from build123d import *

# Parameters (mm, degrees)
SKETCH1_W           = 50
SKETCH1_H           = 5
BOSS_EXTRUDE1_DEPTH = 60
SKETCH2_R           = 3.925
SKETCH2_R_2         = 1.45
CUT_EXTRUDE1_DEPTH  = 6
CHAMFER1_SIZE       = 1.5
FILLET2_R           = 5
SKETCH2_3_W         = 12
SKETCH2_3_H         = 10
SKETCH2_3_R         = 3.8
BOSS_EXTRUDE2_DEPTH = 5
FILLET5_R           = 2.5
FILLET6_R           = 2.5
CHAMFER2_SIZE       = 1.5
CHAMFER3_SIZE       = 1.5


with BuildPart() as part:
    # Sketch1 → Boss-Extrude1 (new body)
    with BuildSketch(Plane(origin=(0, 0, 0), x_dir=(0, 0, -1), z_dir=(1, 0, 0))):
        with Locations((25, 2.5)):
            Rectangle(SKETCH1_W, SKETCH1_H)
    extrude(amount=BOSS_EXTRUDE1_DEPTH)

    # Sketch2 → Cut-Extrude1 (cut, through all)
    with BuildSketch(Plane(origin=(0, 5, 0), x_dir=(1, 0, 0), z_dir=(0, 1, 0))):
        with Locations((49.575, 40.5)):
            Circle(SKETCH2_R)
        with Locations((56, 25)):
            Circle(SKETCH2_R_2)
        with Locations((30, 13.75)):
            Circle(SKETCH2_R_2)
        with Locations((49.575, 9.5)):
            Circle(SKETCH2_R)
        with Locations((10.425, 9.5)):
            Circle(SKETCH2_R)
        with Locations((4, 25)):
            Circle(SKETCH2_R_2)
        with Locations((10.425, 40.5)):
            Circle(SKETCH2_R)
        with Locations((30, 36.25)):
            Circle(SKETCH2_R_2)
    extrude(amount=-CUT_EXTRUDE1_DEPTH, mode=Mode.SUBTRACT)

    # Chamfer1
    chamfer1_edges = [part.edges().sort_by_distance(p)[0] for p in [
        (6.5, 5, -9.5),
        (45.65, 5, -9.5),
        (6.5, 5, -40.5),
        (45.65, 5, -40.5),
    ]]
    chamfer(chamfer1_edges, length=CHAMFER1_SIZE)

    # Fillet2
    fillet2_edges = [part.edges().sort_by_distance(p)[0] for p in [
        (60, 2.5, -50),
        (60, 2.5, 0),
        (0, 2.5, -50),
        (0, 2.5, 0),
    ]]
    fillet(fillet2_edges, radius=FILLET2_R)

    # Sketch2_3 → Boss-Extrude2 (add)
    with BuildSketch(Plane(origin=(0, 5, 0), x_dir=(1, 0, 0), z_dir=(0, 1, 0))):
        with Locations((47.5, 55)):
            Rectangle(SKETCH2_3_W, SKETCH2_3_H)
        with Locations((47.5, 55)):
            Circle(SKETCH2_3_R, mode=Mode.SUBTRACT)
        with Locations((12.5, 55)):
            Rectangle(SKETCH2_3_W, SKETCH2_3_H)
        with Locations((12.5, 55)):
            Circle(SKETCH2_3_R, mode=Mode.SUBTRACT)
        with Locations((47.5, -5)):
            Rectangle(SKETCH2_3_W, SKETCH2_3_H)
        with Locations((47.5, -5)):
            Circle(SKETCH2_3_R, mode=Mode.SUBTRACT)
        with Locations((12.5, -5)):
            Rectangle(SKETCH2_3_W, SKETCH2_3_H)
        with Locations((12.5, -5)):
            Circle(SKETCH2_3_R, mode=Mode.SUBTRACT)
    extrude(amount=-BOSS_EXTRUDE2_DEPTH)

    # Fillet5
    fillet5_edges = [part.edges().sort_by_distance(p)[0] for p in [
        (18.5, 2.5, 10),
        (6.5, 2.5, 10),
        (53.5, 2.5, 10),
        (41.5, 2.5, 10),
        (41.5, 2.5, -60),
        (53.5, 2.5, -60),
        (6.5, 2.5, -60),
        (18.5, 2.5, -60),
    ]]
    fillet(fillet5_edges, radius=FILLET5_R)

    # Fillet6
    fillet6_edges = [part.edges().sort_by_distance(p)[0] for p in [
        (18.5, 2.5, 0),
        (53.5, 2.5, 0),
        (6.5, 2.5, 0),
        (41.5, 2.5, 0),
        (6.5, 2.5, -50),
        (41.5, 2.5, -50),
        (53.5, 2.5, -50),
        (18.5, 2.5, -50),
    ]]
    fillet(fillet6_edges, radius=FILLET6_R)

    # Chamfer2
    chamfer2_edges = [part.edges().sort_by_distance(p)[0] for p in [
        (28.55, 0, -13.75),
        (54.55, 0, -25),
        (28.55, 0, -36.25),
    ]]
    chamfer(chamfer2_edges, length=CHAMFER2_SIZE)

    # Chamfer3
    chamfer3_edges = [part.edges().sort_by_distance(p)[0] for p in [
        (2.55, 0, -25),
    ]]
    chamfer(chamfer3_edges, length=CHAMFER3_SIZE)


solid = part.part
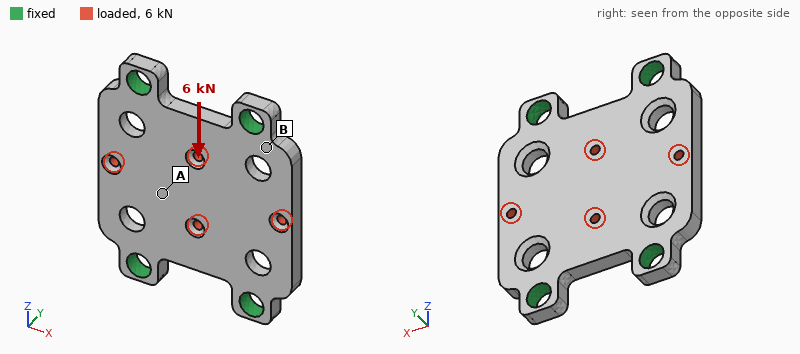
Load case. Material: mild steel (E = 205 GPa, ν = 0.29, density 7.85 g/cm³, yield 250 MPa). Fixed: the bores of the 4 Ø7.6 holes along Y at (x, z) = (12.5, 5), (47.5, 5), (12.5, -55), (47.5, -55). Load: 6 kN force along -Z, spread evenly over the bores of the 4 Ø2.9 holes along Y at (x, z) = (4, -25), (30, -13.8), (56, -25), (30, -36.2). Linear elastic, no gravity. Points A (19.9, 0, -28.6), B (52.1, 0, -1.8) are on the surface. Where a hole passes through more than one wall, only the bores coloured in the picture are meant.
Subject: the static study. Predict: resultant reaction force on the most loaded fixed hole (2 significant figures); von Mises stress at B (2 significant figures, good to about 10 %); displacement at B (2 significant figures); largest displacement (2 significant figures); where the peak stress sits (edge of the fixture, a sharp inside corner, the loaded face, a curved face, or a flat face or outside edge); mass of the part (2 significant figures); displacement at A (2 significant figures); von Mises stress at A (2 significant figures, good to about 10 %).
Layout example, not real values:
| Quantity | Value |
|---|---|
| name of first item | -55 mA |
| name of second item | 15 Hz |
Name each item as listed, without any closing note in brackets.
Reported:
| Quantity | Value |
|---|---|
| resultant reaction force on the most loaded fixed hole | 1.5 kN |
| von Mises stress at B | 22 MPa |
| displacement at B | 0.70 µm |
| largest displacement | 3.6 µm |
| where the peak stress sits | the loaded face |
| mass of the part | 120 g |
| displacement at A | 2.0 µm |
| von Mises stress at A | 6.5 MPa |
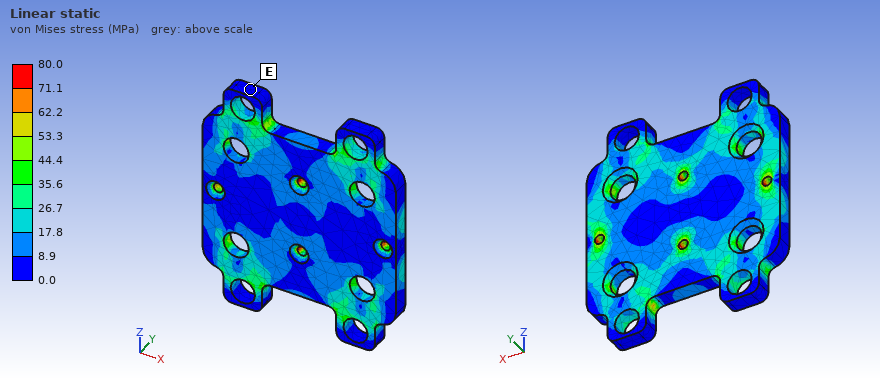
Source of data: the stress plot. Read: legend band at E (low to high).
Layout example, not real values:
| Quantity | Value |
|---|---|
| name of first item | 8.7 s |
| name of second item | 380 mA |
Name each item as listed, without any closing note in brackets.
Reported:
| Quantity | Value |
|---|---|
| legend band at E | 0.0 to 8.9 MPa |
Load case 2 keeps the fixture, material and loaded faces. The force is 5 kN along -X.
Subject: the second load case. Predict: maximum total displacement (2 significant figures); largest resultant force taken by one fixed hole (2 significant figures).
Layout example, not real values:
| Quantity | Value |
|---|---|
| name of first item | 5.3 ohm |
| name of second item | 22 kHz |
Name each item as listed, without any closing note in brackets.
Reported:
| Quantity | Value |
|---|---|
| maximum total displacement | 7.6 µm |
| largest resultant force taken by one fixed hole | 1.3 kN |
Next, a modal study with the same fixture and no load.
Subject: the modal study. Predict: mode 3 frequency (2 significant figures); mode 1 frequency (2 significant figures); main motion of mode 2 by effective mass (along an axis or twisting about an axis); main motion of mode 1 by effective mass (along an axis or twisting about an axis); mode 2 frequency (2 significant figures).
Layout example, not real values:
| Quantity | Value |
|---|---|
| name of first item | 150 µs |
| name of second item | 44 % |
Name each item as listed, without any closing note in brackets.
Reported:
| Quantity | Value |
|---|---|
| mode 3 frequency | 11 kHz |
| mode 1 frequency | 6700 Hz |
| main motion of mode 2 by effective mass | twisting about Z |
| main motion of mode 1 by effective mass | along Y |
| mode 2 frequency | 7900 Hz |
